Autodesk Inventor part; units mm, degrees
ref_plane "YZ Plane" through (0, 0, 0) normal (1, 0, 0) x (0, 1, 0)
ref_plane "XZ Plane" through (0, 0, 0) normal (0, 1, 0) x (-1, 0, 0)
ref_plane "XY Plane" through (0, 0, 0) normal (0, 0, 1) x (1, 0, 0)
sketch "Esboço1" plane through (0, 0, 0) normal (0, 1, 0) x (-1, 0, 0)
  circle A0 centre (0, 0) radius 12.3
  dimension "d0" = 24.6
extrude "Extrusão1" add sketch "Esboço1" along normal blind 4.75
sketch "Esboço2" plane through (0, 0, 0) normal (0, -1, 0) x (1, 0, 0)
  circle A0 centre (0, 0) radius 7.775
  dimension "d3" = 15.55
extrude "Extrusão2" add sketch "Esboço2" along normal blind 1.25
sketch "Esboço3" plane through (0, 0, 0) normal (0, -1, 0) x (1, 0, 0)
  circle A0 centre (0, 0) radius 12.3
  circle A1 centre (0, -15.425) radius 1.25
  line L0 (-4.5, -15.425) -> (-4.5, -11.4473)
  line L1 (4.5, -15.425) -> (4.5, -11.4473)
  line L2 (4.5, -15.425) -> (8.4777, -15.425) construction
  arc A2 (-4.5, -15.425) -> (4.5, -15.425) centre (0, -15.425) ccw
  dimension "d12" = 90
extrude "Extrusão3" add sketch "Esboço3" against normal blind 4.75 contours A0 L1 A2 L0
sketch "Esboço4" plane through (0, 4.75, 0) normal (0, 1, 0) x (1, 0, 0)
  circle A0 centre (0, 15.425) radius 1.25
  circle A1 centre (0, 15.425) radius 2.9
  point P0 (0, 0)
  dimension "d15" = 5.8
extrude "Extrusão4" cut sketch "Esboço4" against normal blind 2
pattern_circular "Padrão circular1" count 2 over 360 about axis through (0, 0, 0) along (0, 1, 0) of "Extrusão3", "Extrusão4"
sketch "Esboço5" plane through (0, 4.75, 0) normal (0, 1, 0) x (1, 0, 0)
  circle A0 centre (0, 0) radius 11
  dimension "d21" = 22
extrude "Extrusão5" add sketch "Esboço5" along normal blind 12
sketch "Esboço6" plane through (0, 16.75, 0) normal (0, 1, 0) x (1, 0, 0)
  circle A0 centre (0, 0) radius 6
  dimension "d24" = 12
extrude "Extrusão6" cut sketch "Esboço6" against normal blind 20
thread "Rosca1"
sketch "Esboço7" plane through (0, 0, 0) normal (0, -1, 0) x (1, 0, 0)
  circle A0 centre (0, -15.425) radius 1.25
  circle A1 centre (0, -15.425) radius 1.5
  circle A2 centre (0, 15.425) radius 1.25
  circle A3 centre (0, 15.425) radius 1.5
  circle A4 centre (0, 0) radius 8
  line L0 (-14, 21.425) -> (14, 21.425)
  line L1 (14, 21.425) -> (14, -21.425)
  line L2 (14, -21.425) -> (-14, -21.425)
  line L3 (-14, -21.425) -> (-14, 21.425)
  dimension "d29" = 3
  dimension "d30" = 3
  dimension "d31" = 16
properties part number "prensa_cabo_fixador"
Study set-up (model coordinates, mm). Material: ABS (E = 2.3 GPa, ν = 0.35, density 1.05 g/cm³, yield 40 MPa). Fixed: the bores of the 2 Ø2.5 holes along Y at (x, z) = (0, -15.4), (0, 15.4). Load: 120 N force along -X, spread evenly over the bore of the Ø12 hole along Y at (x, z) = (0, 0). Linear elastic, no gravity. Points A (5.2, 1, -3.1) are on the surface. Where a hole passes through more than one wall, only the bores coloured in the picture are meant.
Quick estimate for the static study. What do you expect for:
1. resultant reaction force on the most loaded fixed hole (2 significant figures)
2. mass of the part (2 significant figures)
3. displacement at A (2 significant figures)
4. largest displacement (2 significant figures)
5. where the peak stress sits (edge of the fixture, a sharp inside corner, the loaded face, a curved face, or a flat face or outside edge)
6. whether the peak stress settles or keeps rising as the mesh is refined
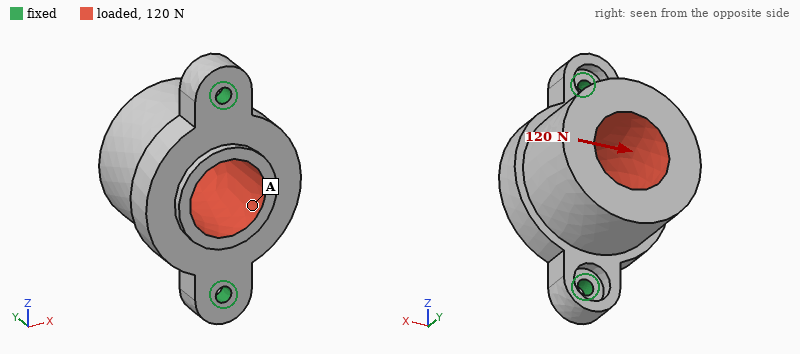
60 N
5.8 g
0.10 mm
0.39 mm
edge of the fixture
keeps rising
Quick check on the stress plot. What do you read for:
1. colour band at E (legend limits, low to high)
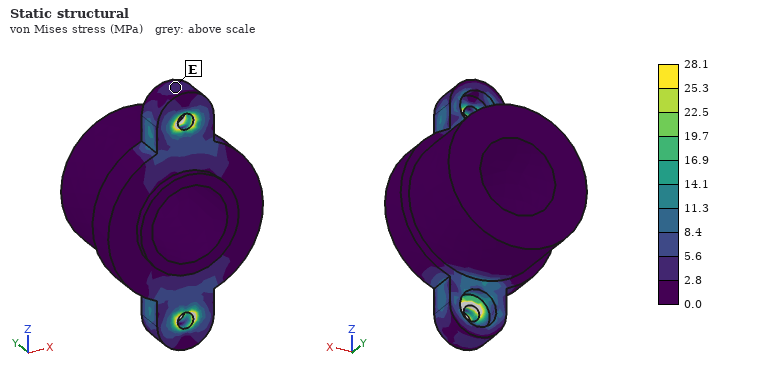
2.8 to 5.6 MPa
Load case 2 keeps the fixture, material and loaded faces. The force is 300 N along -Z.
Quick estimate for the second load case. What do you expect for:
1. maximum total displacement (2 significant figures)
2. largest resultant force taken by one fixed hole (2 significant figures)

51 µm
160 N
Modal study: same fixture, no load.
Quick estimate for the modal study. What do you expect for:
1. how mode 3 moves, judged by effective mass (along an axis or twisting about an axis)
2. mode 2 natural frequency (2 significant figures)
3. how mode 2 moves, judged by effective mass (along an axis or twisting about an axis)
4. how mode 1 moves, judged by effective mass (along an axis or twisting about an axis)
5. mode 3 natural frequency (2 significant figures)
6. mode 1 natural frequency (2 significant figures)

along Z
4200 Hz
along Y
along X
5900 Hz
1300 Hz
